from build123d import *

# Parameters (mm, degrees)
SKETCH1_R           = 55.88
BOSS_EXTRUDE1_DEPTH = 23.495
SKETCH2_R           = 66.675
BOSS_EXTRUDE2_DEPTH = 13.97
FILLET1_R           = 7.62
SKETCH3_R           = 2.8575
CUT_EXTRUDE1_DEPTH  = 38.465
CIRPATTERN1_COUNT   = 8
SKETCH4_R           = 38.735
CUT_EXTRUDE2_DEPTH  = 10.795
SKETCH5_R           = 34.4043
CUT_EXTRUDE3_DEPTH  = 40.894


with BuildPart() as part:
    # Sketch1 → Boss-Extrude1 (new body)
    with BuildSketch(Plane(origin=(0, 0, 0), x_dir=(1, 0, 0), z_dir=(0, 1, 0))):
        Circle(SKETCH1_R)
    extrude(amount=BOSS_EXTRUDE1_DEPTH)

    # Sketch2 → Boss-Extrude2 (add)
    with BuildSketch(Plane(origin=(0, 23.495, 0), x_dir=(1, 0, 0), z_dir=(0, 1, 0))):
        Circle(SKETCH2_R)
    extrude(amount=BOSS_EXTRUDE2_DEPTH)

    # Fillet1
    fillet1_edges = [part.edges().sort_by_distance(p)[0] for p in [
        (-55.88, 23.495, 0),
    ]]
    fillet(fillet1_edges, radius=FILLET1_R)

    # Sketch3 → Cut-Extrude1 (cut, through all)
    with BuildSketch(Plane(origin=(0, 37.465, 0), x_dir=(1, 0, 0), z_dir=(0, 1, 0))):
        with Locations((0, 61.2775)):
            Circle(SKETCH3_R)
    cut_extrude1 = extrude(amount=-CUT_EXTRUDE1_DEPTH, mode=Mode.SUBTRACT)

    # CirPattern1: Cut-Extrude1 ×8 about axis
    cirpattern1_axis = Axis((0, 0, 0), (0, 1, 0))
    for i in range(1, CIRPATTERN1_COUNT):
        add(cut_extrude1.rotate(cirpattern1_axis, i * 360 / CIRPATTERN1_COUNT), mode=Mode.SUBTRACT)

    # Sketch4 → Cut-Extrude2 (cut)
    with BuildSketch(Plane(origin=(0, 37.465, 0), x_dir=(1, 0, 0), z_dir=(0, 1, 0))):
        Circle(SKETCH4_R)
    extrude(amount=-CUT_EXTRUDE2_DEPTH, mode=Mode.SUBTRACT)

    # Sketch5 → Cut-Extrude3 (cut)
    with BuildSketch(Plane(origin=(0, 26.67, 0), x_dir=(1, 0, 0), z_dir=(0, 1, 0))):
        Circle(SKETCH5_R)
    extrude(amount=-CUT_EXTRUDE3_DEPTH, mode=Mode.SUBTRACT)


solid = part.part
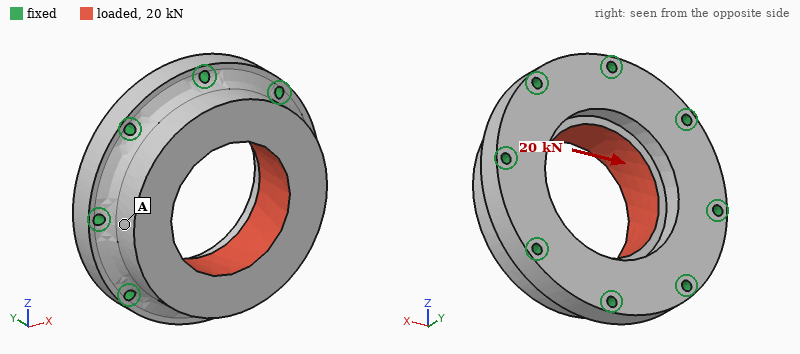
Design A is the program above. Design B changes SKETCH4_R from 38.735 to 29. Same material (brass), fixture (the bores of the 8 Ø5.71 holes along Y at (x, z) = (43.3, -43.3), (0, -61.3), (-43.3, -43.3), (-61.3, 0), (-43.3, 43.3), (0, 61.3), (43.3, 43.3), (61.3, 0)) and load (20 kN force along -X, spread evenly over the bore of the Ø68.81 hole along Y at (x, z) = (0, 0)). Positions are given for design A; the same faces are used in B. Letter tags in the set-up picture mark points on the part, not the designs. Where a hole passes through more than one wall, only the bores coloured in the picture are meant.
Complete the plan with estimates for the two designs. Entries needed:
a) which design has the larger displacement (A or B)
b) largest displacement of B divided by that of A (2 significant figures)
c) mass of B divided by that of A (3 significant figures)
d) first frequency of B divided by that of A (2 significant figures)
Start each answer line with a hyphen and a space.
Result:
- A
- 0.91
- 1.08
- 0.92
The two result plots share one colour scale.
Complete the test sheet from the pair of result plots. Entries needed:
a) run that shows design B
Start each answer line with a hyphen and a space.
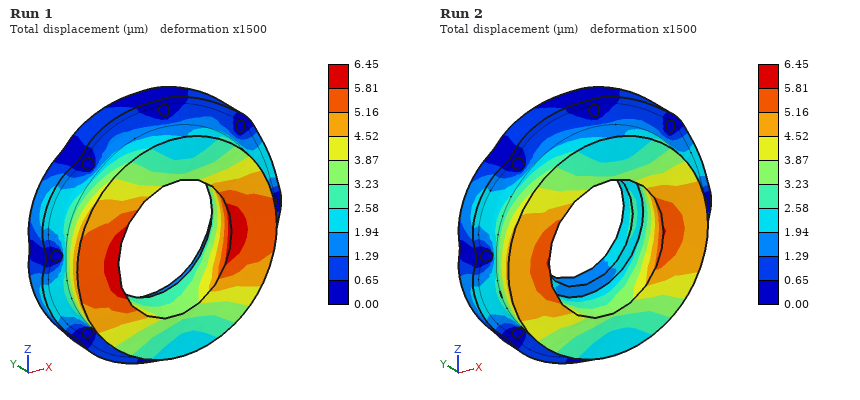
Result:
- Run 2
